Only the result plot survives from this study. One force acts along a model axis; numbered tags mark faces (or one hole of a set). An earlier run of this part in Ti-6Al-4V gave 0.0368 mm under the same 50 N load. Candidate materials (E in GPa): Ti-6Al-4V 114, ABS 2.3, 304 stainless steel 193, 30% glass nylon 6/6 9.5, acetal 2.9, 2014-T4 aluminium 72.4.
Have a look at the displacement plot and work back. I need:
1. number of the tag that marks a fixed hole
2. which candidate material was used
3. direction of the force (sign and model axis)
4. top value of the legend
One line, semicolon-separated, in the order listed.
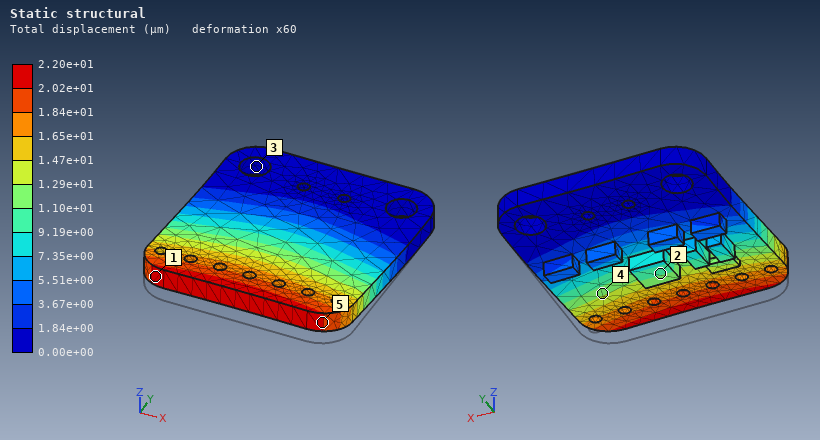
3; 304 stainless steel; +Z; 2.20e+01 µm
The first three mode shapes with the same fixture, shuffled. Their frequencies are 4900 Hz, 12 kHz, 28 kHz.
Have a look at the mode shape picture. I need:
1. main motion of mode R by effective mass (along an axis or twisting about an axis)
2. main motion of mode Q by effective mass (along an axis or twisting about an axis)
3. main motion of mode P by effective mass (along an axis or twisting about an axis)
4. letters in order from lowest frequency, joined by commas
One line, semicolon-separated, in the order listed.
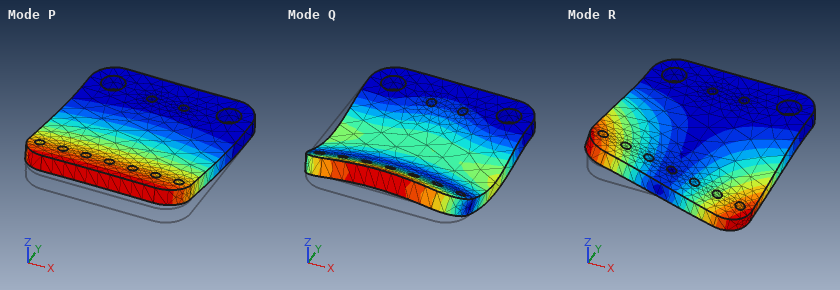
twisting about Y; along Z; along Z; P, R, Q
